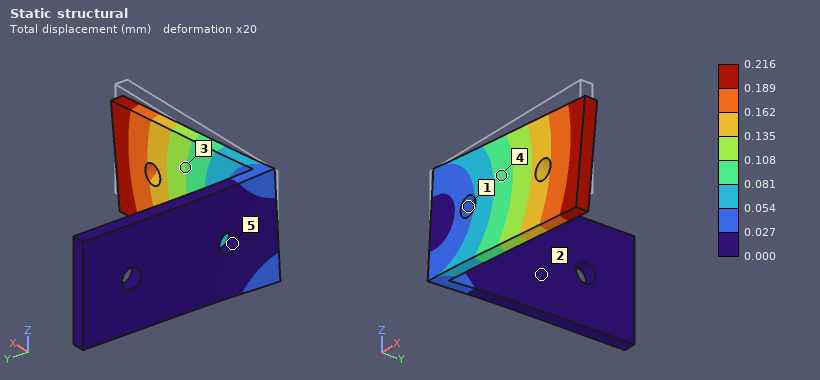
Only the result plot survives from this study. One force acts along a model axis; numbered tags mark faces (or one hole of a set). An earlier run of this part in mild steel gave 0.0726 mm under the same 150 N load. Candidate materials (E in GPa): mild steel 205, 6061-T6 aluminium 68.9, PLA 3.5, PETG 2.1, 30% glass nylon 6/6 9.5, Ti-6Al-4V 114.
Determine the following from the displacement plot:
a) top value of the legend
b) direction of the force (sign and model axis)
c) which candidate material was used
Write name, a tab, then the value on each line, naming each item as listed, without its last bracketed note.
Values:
top value of the legend	0.216 mm
direction of the force	-Z
which candidate material was used	6061-T6 aluminium
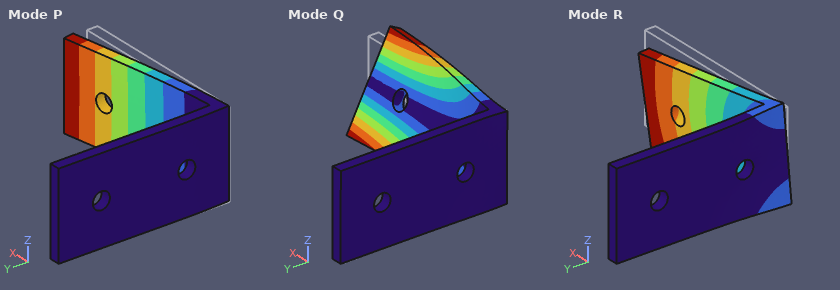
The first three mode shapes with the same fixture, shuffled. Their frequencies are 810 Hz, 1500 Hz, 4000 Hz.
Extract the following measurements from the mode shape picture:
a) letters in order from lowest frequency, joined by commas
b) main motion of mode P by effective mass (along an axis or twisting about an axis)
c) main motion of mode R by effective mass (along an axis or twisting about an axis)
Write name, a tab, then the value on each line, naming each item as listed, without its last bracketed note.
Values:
letters in order from lowest frequency, joined by commas	P, R, Q
main motion of mode P by effective mass	along Y
main motion of mode R by effective mass	along Z
